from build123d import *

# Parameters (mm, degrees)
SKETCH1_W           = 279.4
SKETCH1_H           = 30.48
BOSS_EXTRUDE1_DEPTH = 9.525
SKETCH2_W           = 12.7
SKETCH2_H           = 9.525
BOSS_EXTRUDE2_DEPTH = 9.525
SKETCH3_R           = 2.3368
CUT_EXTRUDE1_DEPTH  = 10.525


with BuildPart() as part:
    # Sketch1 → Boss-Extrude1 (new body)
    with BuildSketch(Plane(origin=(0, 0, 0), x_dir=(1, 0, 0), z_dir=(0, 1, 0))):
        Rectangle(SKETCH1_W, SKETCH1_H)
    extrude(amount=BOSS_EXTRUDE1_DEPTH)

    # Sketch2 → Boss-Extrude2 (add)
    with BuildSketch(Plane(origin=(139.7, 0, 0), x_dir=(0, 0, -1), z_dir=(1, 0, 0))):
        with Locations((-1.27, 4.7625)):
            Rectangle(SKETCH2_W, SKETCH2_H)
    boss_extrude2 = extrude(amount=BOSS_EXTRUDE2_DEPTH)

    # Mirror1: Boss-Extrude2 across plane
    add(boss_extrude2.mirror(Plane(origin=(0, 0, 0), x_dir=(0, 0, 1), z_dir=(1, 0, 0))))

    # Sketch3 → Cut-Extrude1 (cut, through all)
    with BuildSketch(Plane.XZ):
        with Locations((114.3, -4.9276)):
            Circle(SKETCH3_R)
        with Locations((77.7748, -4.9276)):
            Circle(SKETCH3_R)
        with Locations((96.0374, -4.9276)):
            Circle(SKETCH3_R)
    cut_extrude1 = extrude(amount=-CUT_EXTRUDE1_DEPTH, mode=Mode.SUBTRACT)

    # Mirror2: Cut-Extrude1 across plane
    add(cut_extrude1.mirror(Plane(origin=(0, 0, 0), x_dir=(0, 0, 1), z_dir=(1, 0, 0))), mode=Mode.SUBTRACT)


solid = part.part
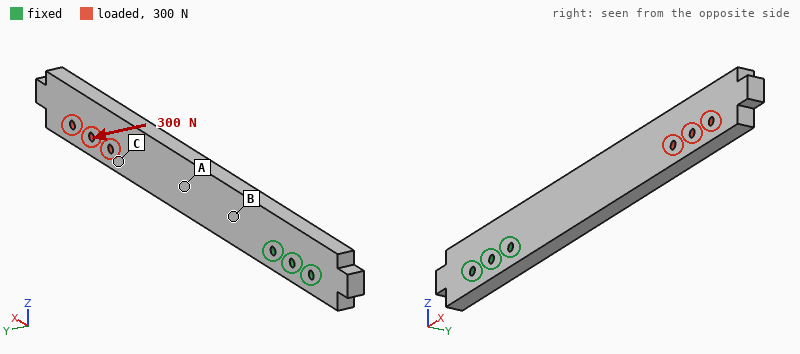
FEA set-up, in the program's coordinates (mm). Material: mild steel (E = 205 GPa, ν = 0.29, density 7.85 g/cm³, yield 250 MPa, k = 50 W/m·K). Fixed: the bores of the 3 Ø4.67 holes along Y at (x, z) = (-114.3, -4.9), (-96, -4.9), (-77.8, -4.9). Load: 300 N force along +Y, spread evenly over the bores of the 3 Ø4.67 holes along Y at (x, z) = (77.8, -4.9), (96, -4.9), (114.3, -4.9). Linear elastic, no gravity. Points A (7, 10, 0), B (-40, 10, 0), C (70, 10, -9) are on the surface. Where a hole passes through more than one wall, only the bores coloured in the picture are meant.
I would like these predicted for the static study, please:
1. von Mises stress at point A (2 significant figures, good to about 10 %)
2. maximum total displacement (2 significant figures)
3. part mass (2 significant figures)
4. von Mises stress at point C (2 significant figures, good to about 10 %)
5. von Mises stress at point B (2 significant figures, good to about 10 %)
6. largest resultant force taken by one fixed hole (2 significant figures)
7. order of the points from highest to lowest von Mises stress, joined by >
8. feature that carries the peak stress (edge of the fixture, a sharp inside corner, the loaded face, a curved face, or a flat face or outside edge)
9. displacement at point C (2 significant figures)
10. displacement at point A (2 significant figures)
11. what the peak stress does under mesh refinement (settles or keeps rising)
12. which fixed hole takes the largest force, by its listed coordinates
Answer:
58 MPa
1.8 mm
650 g
18 MPa
88 MPa
1.4 kN
B > A > C
edge of the fixture
0.94 mm
0.37 mm
keeps rising
(-77.8, -4.9)
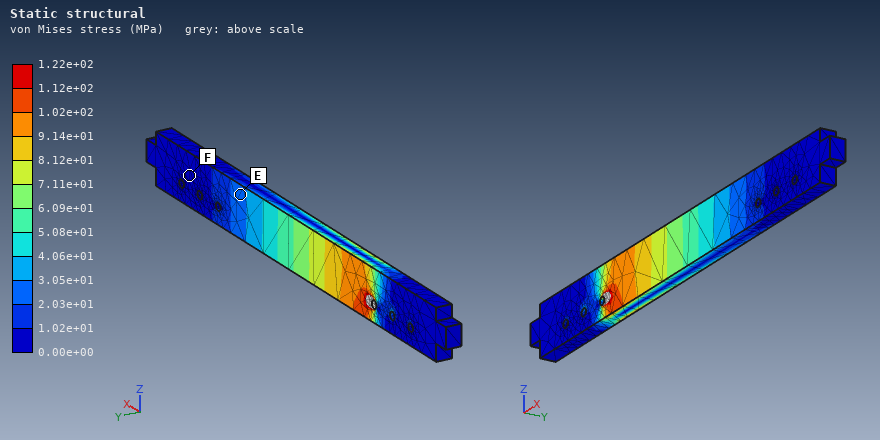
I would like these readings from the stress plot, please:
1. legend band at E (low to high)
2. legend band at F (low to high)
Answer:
2.03e+01 to 3.05e+01 MPa
0.00e+00 to 1.02e+01 MPa
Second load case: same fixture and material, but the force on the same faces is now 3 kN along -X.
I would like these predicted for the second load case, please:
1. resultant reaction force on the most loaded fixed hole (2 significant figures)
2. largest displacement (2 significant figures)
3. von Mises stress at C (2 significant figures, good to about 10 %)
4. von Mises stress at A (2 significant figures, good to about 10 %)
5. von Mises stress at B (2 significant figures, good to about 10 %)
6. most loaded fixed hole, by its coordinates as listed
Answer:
2.4 kN
79 µm
17 MPa
10 MPa
10 MPa
(-77.8, -4.9)
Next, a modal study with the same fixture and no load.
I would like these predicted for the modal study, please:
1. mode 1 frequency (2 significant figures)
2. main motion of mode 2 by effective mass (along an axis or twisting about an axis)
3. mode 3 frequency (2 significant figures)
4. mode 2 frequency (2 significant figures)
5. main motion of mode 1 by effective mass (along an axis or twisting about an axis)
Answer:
160 Hz
along Z
970 Hz
460 Hz
along Y
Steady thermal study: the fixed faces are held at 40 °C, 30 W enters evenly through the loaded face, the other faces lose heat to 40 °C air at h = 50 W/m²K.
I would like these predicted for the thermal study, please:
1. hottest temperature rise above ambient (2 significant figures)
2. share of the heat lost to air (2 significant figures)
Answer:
69 K
94 %
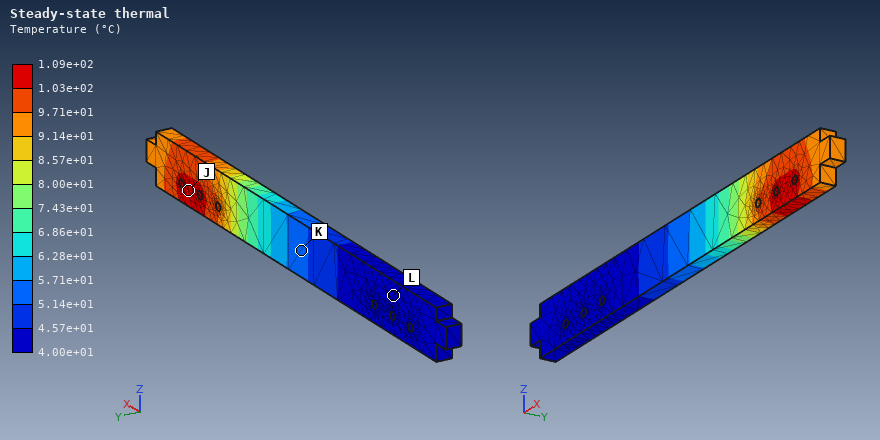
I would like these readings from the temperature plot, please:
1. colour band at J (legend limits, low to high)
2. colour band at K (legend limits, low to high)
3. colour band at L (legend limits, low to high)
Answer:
1.03e+02 to 1.09e+02 °C
5.14e+01 to 5.71e+01 °C
4.00e+01 to 4.57e+01 °C
